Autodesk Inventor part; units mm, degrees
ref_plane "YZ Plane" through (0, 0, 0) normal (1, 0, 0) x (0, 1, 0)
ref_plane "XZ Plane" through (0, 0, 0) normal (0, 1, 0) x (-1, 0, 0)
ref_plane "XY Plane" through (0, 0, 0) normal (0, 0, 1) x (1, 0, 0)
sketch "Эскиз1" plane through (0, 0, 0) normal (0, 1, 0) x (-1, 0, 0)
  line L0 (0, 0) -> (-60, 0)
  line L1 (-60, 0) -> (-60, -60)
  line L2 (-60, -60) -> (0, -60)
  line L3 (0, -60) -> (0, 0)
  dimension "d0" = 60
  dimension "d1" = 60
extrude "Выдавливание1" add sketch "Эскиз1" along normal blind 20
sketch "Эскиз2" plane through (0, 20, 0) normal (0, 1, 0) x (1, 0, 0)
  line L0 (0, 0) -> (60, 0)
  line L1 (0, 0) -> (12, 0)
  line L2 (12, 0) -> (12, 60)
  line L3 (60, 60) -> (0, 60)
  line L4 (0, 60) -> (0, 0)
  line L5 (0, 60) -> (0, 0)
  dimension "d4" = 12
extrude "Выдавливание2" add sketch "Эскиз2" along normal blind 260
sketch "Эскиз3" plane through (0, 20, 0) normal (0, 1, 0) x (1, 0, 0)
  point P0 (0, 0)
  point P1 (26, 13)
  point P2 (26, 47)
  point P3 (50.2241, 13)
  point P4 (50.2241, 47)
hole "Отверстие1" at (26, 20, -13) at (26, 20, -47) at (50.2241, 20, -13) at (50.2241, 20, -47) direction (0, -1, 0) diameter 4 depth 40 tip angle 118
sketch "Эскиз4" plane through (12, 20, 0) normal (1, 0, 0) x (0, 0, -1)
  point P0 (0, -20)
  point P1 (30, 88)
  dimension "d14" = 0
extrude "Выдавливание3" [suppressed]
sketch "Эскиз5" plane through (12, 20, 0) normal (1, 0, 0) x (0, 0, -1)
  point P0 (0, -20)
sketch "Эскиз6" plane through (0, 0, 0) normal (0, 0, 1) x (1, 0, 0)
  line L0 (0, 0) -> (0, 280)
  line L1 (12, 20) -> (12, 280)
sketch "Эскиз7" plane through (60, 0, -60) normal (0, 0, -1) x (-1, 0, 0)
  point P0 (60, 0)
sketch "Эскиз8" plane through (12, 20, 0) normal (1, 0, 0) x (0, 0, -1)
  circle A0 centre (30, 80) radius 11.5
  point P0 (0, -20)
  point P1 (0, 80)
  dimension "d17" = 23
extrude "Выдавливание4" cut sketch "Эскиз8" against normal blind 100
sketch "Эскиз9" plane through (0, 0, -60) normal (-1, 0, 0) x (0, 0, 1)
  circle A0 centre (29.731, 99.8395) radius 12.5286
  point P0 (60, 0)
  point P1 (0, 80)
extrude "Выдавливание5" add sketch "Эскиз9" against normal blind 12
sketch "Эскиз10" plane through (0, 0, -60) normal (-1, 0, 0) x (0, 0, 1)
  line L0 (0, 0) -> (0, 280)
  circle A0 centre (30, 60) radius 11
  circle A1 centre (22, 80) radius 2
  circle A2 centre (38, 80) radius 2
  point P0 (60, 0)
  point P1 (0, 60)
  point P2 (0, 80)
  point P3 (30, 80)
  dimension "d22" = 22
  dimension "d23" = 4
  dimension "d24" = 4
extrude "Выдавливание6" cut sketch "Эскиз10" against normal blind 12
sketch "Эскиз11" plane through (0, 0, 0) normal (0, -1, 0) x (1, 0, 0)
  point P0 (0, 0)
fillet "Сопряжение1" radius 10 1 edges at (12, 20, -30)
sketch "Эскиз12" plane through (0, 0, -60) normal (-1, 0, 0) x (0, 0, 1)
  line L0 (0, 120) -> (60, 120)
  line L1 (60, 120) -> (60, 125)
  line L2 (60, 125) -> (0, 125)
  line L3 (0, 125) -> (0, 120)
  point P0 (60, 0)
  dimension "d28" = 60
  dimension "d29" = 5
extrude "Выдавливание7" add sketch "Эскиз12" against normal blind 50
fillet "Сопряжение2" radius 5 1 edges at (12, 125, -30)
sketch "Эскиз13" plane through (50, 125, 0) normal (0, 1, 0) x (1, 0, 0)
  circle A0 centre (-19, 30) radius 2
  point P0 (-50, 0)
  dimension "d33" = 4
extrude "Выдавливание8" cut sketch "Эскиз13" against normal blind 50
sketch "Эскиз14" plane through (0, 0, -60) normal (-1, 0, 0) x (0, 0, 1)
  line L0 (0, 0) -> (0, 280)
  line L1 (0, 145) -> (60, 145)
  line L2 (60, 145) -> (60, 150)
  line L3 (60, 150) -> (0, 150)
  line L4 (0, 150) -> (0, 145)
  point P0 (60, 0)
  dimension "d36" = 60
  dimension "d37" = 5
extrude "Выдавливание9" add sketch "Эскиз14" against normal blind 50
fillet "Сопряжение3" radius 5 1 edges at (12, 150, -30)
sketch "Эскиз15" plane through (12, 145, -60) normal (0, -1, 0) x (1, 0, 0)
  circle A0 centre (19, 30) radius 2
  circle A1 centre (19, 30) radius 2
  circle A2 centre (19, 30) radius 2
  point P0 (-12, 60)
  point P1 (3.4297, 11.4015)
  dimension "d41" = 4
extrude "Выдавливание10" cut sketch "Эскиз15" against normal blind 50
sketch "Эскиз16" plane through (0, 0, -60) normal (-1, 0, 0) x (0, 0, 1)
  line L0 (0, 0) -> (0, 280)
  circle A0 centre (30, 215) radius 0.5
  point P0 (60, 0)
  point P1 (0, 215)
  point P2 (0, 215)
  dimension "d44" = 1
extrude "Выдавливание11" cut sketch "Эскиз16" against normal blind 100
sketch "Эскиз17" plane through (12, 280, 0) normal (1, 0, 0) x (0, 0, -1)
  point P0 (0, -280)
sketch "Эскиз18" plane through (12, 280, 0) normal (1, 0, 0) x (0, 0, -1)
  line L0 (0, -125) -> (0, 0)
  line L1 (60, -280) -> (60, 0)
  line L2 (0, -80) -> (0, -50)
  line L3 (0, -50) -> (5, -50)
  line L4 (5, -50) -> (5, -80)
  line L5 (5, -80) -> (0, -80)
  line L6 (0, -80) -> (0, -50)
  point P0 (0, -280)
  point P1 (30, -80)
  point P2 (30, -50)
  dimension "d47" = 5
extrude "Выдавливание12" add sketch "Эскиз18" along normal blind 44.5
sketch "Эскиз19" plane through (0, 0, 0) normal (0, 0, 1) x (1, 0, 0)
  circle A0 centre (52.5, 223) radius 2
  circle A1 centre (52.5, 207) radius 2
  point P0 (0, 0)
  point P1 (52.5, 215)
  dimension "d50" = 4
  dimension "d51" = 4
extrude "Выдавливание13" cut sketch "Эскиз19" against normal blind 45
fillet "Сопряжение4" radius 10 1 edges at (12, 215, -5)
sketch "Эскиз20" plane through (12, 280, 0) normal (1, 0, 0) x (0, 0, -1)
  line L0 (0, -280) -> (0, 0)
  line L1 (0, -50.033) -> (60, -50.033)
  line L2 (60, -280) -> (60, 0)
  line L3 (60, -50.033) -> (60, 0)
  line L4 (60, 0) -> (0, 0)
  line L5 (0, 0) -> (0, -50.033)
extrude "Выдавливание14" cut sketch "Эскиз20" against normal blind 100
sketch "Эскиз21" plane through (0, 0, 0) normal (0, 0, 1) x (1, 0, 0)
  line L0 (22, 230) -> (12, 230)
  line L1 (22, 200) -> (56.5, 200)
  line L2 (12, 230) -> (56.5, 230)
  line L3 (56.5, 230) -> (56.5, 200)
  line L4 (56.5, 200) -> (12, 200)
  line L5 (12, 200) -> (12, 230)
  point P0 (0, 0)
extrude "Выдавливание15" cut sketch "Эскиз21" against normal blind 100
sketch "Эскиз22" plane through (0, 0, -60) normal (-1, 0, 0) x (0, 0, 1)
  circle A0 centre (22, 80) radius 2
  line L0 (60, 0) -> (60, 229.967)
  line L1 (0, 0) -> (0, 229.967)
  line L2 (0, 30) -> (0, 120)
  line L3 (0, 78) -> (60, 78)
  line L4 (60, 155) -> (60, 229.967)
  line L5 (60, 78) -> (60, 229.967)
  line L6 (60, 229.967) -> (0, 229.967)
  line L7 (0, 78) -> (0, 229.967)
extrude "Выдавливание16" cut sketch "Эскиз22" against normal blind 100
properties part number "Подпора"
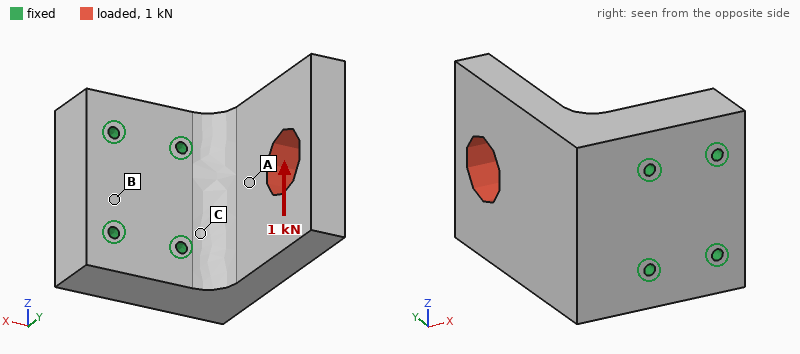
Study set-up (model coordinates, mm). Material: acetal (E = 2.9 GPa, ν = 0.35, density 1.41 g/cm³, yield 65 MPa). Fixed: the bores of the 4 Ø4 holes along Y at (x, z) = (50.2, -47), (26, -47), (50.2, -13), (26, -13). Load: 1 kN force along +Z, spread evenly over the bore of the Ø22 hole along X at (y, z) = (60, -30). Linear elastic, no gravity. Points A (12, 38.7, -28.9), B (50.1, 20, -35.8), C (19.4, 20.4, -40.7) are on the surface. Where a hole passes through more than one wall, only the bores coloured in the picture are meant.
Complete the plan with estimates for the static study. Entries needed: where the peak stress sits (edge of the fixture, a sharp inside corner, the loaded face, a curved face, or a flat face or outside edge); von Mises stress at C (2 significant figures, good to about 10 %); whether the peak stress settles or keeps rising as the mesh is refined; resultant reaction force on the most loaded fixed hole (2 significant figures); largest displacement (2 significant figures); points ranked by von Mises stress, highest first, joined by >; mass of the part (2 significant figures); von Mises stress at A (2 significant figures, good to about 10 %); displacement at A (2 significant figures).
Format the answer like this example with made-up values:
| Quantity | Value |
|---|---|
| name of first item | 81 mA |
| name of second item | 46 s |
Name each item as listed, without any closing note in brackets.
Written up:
| Quantity | Value |
|---|---|
| where the peak stress sits | edge of the fixture |
| von Mises stress at C | 9.2 MPa |
| whether the peak stress settles or keeps rising as the mesh is refined | keeps rising |
| resultant reaction force on the most loaded fixed hole | 1.2 kN |
| largest displacement | 0.49 mm |
| points ranked by von Mises stress, highest first, joined by > | C > A > B |
| mass of the part | 150 g |
| von Mises stress at A | 6.1 MPa |
| displacement at A | 0.17 mm |
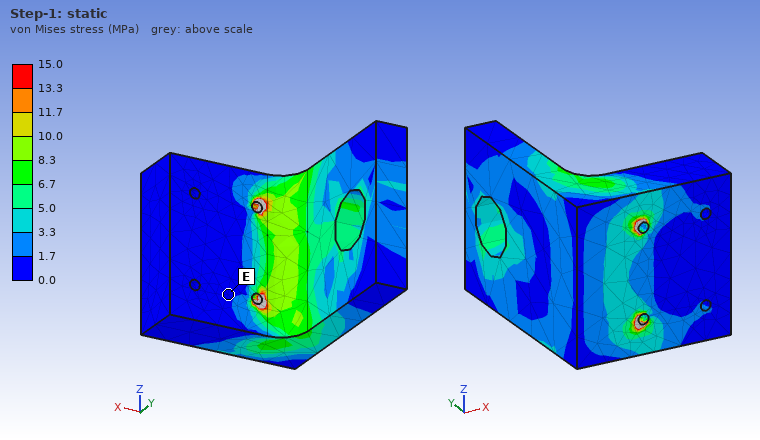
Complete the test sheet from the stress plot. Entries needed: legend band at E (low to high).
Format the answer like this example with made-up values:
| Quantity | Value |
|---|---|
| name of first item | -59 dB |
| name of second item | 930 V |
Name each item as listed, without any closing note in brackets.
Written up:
| Quantity | Value |
|---|---|
| legend band at E | 0.0 to 1.7 MPa |
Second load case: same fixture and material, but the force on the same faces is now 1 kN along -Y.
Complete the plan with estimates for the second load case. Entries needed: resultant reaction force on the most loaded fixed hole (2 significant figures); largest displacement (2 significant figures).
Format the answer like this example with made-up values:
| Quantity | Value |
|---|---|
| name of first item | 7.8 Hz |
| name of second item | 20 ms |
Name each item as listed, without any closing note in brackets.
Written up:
| Quantity | Value |
|---|---|
| resultant reaction force on the most loaded fixed hole | 600 N |
| largest displacement | 0.24 mm |
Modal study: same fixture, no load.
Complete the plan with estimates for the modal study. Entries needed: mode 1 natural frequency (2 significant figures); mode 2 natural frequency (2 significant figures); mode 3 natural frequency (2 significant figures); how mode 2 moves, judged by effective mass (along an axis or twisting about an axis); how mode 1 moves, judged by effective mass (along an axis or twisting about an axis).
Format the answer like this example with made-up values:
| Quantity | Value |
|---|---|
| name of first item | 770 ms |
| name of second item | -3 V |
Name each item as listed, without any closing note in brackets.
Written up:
| Quantity | Value |
|---|---|
| mode 1 natural frequency | 730 Hz |
| mode 2 natural frequency | 1300 Hz |
| mode 3 natural frequency | 1600 Hz |
| how mode 2 moves, judged by effective mass | along Z |
| how mode 1 moves, judged by effective mass | along X |
